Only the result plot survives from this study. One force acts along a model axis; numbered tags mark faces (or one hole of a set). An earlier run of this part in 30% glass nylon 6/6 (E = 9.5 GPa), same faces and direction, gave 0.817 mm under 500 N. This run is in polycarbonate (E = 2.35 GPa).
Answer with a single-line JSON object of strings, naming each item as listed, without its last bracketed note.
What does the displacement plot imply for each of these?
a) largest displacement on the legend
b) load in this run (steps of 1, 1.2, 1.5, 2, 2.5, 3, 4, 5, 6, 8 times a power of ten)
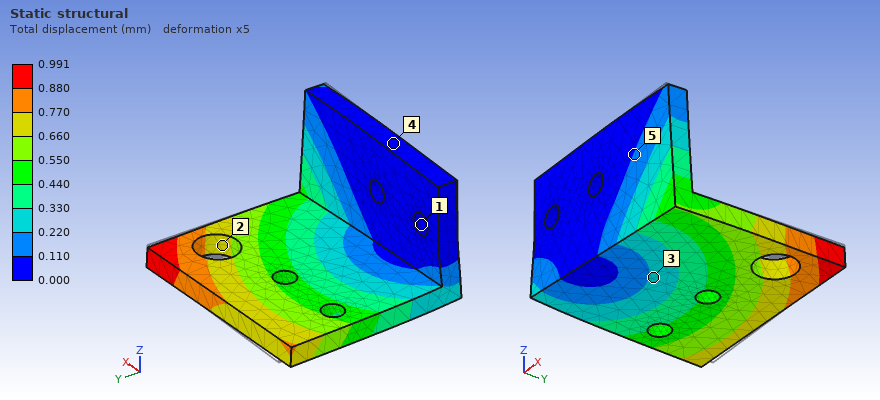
{"largest displacement on the legend": "0.991 mm", "load in this run": "150 N"}
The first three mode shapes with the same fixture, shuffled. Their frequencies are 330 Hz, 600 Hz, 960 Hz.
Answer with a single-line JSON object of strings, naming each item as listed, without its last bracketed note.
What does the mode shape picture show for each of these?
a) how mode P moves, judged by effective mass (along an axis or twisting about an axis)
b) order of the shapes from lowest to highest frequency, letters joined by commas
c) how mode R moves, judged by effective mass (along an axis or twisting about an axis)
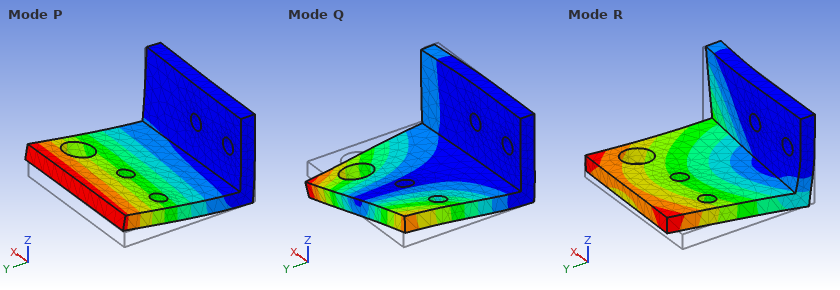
{"how mode P moves, judged by effective mass": "along Z", "order of the shapes from lowest to highest frequency, letters joined by commas": "P, R, Q", "how mode R moves, judged by effective mass": "along X"}
